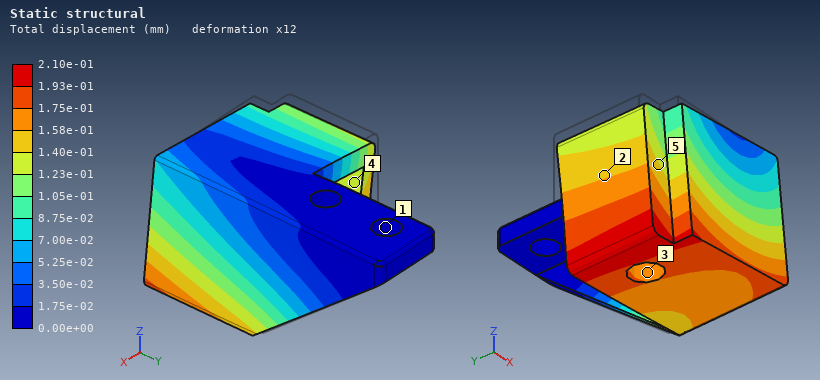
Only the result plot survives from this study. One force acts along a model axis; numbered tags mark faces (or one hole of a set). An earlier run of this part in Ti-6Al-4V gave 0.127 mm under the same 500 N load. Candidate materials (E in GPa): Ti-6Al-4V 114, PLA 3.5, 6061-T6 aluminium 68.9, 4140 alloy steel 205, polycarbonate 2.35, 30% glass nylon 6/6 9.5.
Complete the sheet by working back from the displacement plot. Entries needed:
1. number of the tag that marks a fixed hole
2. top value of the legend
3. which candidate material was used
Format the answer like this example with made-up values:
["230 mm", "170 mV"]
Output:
["1", "2.10e-01 mm", "6061-T6 aluminium"]
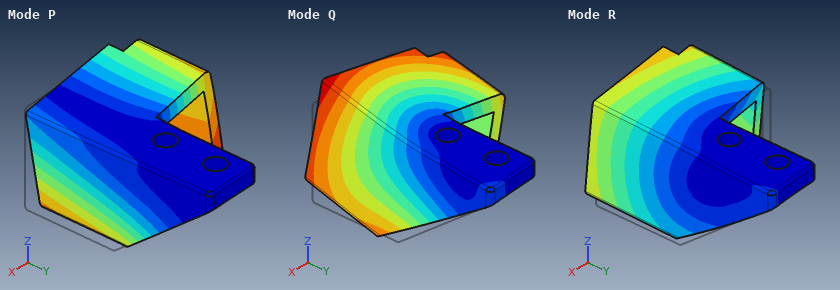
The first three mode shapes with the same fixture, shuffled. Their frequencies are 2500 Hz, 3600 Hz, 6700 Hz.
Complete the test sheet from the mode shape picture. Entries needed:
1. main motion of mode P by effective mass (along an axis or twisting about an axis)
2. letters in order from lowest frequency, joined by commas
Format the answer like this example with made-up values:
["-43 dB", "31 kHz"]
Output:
["along X", "P, R, Q"]
